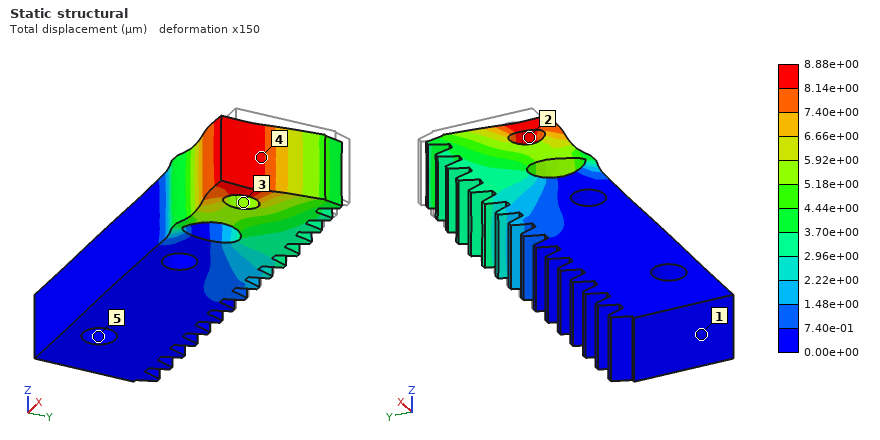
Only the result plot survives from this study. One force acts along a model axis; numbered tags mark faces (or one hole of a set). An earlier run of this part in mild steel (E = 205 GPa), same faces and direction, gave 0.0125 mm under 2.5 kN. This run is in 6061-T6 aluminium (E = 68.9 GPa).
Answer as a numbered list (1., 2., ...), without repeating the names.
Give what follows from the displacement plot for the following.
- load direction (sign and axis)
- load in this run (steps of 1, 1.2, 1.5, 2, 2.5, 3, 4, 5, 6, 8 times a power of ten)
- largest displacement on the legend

1. -X
2. 600 N
3. 8.88e+00 µm
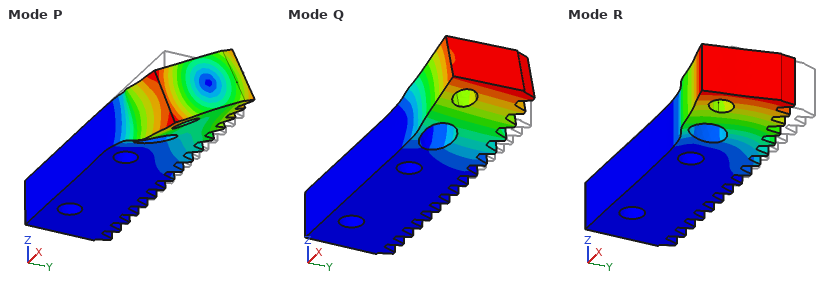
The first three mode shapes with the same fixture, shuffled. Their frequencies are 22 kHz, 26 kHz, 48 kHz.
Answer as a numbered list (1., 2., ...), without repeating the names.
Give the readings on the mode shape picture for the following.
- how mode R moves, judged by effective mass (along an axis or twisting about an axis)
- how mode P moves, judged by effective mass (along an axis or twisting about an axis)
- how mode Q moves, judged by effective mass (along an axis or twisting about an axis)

1. along Y
2. twisting about X
3. along Z
